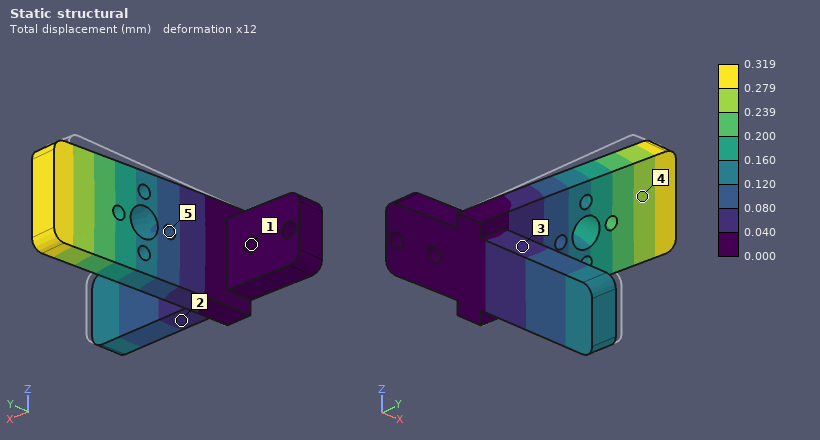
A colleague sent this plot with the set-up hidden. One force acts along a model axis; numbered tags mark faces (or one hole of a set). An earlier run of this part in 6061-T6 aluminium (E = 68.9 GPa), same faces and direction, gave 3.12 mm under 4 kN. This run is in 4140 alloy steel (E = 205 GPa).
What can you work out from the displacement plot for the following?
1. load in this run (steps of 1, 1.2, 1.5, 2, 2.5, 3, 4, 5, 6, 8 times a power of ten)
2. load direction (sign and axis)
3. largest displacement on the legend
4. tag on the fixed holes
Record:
1.2 kN
+X
0.319 mm
1
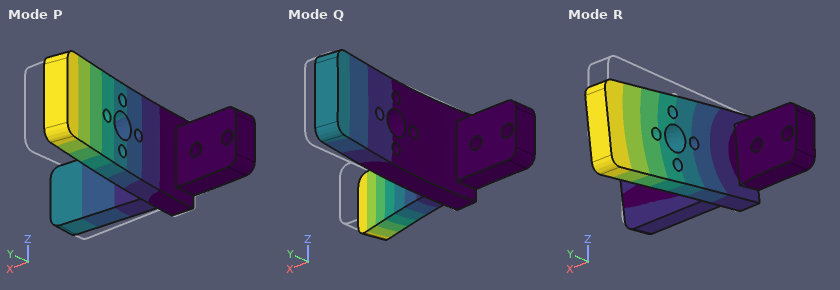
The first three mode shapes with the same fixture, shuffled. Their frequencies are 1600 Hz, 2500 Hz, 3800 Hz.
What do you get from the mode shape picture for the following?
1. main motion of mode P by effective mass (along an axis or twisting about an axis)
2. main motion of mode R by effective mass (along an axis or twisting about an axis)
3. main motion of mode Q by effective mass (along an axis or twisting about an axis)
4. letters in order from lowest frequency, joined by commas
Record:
along X
along Z
along Y
P, R, Q
